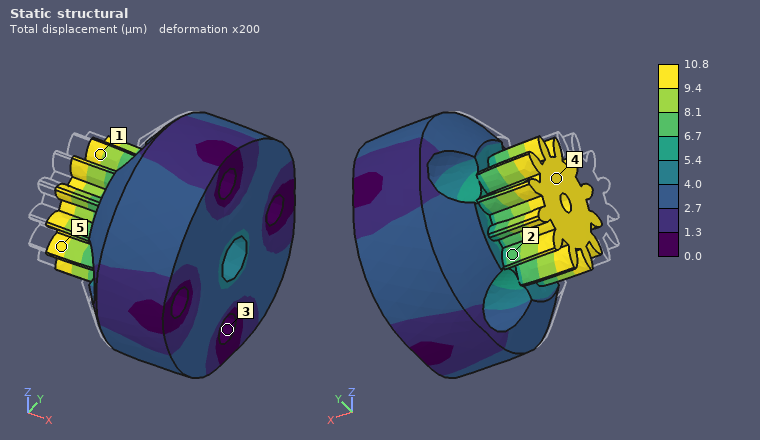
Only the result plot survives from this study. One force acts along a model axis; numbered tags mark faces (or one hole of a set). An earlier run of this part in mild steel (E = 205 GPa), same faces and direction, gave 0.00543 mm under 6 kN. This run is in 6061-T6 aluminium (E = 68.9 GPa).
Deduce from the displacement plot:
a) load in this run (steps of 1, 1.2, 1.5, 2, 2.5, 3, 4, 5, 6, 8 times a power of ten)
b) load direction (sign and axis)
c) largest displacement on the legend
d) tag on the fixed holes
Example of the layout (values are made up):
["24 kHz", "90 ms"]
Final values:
["4 kN", "+X", "10.8 µm", "3"]
